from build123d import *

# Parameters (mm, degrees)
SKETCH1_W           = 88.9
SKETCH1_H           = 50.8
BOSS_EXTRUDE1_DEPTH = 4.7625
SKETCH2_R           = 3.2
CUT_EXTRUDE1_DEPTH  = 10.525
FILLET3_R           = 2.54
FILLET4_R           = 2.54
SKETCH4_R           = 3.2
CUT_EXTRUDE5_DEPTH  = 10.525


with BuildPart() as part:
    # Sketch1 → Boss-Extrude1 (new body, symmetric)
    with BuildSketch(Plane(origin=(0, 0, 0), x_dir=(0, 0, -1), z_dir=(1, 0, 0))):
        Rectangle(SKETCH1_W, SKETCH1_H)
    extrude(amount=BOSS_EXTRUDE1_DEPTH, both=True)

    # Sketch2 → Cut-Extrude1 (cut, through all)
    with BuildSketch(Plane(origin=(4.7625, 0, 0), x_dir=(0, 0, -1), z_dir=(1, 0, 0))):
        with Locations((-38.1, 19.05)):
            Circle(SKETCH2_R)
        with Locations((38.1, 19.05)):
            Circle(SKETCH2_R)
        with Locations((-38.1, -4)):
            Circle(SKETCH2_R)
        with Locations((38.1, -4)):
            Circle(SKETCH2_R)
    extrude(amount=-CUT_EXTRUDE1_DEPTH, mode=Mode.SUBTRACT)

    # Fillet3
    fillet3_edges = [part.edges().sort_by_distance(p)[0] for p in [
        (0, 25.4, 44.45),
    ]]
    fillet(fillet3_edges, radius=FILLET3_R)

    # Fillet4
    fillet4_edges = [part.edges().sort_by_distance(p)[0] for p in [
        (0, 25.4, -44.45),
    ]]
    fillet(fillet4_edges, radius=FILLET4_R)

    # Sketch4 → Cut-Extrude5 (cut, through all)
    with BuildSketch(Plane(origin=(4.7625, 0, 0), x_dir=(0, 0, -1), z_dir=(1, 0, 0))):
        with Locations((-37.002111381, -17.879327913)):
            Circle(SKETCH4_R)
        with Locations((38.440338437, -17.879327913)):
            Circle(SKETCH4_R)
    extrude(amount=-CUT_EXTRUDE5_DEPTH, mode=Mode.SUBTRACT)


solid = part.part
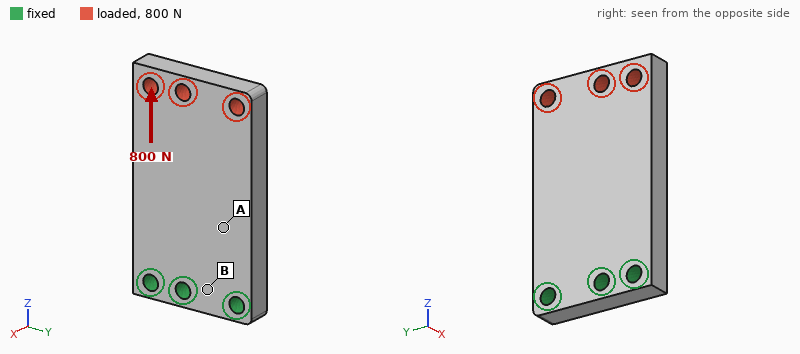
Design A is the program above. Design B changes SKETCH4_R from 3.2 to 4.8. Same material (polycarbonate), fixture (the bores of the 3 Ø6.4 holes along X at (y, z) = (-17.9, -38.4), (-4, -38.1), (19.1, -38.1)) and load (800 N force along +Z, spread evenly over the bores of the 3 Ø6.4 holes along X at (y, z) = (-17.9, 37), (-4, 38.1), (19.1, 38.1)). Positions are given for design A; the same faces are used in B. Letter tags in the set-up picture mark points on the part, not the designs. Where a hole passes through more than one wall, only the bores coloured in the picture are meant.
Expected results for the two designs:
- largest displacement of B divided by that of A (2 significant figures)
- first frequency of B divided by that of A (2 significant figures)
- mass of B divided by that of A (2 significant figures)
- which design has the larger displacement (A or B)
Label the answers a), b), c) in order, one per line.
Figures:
a) 1.5
b) 1.0
c) 0.98
d) B
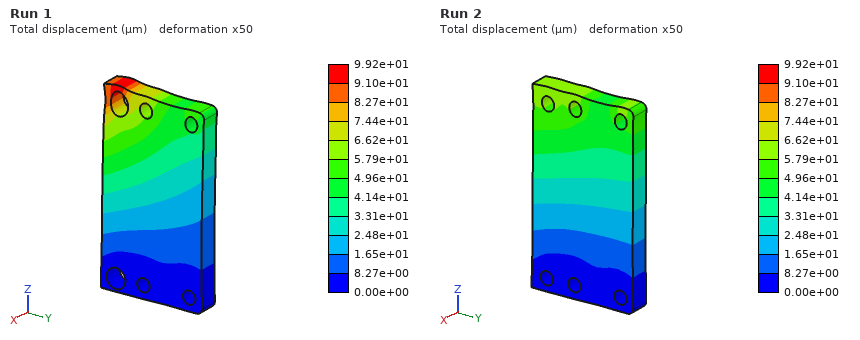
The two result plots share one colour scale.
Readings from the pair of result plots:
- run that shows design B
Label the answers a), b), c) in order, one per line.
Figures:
a) Run 1
